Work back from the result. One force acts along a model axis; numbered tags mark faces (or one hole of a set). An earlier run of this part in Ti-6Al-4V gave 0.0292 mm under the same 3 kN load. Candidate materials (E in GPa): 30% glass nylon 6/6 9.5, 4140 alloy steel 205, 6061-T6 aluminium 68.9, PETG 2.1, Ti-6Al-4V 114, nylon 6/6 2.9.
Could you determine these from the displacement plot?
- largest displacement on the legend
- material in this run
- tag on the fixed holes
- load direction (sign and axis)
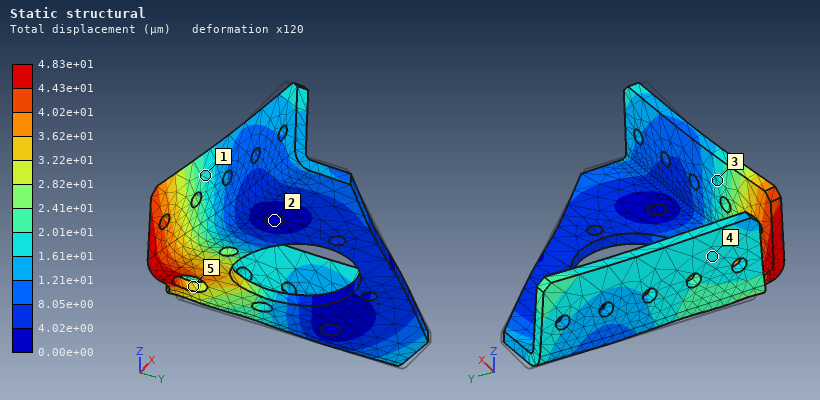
4.83e+01 µm
6061-T6 aluminium
2
-Y
